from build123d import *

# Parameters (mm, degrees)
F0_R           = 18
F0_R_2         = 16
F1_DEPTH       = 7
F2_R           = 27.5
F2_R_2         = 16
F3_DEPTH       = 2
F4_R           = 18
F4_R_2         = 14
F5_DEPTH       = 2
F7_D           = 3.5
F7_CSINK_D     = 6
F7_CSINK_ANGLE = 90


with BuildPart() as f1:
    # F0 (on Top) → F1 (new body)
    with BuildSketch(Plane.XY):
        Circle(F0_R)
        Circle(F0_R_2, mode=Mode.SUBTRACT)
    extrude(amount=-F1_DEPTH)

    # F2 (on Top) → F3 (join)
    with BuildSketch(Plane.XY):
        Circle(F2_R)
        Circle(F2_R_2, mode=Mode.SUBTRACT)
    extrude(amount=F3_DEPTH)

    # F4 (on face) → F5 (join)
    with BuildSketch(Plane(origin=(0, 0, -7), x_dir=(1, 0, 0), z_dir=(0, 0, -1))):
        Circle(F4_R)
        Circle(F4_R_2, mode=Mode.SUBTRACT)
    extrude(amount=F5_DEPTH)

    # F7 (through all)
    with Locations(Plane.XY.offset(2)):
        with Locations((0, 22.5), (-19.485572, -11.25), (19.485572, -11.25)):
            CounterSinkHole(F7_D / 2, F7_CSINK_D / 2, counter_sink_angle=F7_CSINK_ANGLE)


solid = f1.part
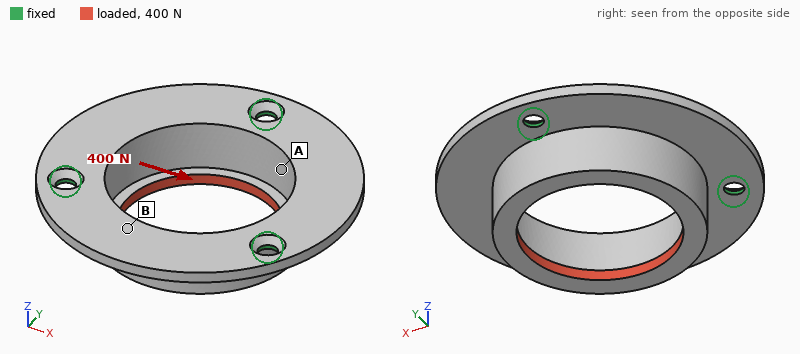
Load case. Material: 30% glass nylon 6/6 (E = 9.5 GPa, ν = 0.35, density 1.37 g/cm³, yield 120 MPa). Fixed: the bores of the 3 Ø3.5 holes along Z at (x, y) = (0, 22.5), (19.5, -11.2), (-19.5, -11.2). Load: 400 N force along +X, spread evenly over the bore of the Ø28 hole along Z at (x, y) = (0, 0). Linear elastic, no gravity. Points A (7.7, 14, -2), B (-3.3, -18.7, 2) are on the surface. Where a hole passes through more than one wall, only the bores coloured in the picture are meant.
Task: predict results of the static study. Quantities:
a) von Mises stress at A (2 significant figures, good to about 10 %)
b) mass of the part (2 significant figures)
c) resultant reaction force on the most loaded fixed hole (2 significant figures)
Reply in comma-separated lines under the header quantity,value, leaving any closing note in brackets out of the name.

quantity,value
von Mises stress at A,8.7 MPa
mass of the part,7.3 g
resultant reaction force on the most loaded fixed hole,160 N
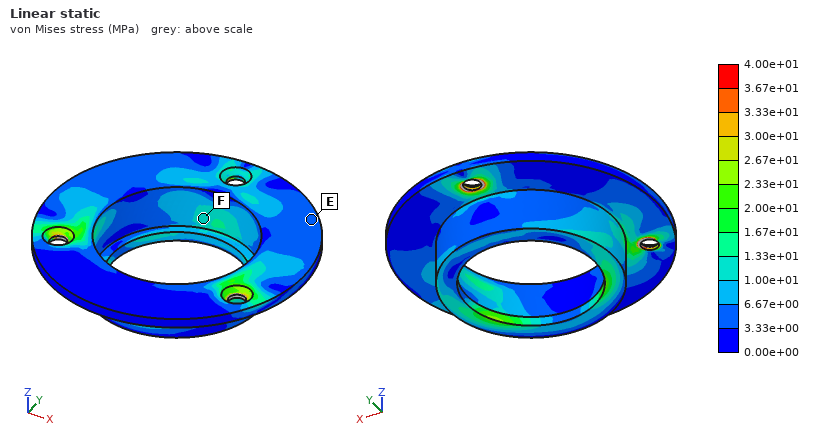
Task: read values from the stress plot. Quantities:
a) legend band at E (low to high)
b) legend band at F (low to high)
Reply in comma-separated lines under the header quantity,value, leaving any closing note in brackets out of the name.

quantity,value
legend band at E,3.33e+00 to 6.67e+00 MPa
legend band at F,1.00e+01 to 1.33e+01 MPa
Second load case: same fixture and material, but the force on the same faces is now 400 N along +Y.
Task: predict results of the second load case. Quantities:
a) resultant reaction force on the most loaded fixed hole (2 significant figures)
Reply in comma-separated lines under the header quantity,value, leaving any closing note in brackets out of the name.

quantity,value
resultant reaction force on the most loaded fixed hole,160 N
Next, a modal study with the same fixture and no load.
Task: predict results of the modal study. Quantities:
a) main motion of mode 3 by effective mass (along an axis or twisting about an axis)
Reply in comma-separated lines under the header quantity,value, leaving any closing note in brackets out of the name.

quantity,value
main motion of mode 3 by effective mass,along Z
